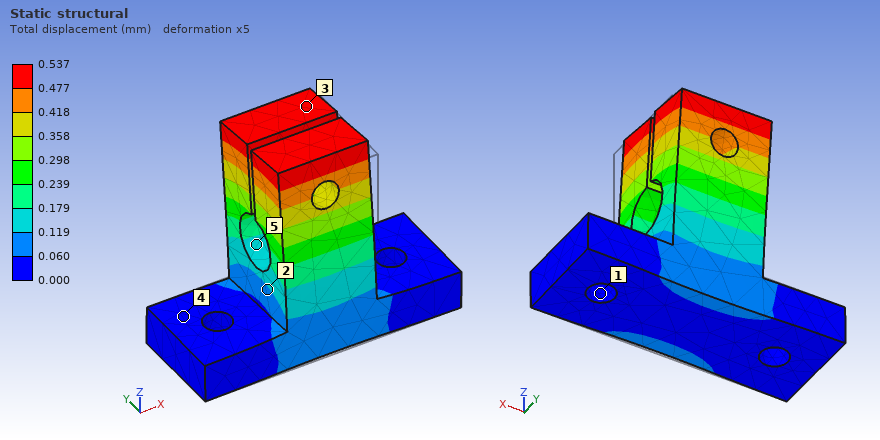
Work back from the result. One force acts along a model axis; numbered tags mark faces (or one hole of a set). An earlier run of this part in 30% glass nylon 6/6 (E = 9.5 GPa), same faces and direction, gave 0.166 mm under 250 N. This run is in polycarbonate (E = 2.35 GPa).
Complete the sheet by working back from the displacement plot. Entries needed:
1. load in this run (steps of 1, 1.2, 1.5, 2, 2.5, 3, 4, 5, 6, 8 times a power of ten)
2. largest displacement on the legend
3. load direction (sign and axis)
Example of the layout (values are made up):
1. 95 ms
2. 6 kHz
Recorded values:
1. 200 N
2. 0.537 mm
3. +Y
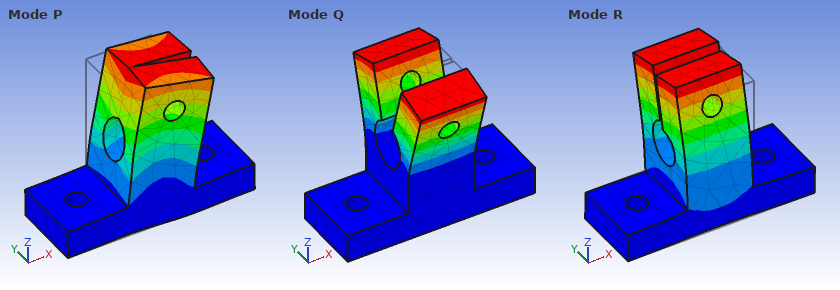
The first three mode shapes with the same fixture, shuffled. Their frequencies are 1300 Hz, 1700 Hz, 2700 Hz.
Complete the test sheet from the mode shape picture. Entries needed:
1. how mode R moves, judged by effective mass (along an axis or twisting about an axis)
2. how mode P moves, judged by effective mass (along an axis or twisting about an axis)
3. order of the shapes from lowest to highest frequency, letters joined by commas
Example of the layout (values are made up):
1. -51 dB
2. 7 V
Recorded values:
1. along Y
2. along X
3. R, Q, P
